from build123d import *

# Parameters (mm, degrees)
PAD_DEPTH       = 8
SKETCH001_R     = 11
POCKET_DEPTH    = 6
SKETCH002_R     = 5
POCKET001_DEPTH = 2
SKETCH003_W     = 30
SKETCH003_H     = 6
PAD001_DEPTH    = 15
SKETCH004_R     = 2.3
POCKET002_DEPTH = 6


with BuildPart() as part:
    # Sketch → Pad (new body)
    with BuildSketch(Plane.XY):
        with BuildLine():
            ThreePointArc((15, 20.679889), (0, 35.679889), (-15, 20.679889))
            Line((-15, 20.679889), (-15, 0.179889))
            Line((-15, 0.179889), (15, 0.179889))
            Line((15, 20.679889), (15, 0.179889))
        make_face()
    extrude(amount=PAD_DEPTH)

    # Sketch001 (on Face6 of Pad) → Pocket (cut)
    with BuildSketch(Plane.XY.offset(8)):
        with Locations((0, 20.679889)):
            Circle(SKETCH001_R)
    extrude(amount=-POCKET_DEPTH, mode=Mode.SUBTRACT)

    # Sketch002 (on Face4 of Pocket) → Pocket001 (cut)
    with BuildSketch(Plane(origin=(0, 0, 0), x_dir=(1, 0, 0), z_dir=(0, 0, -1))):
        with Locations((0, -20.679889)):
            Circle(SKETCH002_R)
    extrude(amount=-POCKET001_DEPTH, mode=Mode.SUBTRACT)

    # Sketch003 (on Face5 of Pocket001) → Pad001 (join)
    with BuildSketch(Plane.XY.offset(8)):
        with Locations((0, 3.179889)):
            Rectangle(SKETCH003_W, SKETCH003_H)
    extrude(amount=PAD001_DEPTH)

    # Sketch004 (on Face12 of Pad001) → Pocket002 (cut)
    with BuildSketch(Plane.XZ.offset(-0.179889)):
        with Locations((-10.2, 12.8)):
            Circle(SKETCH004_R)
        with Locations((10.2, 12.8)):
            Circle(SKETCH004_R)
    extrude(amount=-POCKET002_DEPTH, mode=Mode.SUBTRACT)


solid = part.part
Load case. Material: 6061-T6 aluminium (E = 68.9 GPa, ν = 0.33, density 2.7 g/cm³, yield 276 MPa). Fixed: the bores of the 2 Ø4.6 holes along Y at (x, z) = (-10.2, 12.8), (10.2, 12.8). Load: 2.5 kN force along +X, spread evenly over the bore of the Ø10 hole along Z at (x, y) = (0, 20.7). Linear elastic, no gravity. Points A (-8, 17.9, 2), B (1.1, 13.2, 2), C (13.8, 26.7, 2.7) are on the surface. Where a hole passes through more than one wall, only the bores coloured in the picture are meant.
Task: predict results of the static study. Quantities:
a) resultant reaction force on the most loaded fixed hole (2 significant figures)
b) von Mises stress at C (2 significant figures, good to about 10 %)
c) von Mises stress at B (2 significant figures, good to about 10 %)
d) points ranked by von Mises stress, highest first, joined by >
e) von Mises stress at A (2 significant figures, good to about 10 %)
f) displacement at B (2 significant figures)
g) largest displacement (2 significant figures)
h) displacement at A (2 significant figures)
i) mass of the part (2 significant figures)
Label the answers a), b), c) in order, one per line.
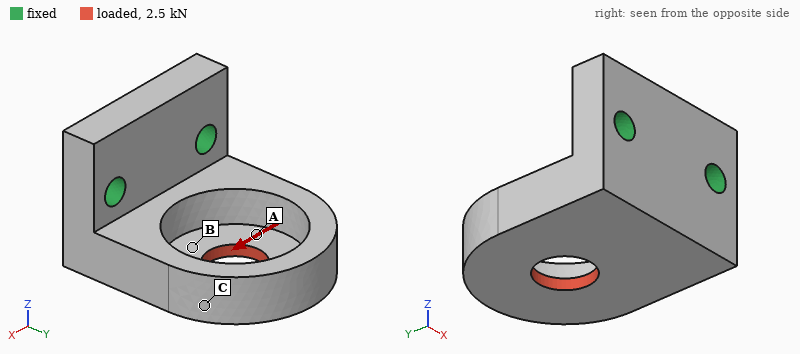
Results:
a) 2.6 kN
b) 28 MPa
c) 110 MPa
d) B > A > C
e) 75 MPa
f) 29 µm
g) 97 µm
h) 47 µm
i) 21 g
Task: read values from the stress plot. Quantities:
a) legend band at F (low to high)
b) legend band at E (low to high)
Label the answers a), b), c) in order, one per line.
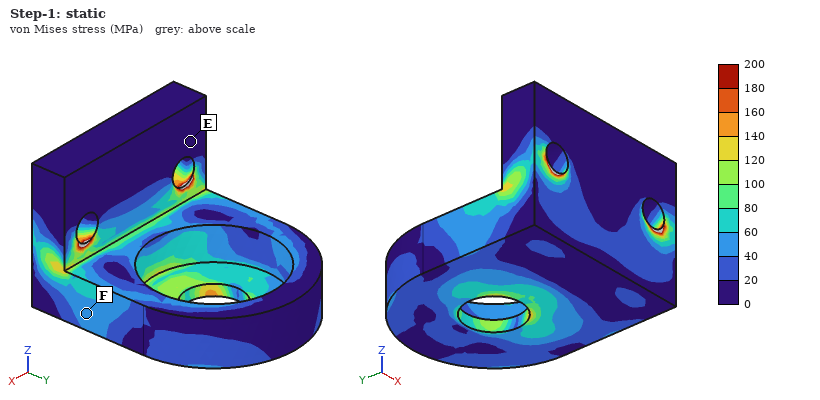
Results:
a) 40 to 60 MPa
b) 0 to 20 MPa
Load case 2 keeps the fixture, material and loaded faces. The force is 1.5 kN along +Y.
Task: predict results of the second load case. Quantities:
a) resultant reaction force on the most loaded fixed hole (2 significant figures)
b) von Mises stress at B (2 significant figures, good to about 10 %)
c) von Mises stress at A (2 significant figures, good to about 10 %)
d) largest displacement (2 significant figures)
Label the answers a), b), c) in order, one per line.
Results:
a) 750 N
b) 22 MPa
c) 29 MPa
d) 0.10 mm
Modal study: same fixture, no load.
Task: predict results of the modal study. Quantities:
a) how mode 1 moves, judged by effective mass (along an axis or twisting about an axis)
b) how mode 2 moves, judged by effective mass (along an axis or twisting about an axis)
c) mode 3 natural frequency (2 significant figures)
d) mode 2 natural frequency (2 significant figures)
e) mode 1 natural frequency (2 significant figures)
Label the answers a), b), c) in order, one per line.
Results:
a) along Z
b) along X
c) 15 kHz
d) 8500 Hz
e) 4600 Hz
